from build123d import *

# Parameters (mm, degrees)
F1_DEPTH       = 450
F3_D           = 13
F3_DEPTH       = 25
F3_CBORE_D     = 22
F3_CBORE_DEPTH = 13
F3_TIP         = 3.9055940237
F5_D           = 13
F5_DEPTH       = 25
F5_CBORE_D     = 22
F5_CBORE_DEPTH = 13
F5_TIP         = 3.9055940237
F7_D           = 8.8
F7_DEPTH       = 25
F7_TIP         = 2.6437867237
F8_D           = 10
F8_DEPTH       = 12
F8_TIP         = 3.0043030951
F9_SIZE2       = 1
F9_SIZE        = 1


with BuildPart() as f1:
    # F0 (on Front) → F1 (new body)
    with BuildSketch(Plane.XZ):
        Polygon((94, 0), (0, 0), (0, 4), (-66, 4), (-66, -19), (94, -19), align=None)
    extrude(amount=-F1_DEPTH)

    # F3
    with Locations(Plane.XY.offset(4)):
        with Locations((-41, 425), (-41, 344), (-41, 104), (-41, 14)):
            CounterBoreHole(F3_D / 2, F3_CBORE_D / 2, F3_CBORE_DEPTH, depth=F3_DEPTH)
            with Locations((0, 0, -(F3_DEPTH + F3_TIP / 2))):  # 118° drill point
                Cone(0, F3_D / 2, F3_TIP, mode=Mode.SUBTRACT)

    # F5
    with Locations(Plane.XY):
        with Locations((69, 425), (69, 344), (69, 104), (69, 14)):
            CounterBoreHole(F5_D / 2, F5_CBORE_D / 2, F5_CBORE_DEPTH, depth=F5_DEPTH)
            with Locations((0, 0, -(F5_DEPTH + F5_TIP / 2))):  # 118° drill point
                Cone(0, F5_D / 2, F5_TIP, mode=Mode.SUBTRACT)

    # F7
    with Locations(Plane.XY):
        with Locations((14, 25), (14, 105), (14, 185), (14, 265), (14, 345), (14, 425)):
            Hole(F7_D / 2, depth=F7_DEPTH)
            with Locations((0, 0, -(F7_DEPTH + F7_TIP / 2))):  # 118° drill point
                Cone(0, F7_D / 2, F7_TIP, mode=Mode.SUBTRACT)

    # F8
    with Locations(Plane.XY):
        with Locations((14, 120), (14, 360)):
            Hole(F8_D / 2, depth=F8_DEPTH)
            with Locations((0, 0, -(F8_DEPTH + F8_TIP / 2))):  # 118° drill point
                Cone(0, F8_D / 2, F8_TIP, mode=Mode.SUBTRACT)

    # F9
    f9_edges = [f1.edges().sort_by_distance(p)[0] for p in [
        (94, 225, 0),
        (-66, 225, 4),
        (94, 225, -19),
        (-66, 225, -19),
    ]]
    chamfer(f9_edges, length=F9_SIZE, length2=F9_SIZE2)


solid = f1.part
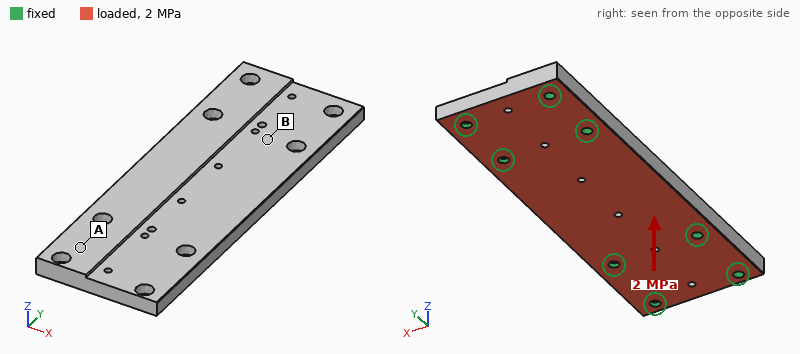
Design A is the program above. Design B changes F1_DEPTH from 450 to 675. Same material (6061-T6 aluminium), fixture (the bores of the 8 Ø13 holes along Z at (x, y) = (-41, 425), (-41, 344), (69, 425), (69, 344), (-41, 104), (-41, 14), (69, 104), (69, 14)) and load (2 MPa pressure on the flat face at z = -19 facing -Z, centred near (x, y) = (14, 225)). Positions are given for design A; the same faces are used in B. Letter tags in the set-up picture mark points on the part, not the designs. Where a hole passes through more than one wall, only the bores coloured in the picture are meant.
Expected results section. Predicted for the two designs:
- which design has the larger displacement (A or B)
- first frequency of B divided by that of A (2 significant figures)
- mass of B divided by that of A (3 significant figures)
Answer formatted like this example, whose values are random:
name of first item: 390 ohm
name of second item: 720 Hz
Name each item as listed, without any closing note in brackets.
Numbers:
which design has the larger displacement: B
first frequency of B divided by that of A: 0.16
mass of B divided by that of A: 1.52
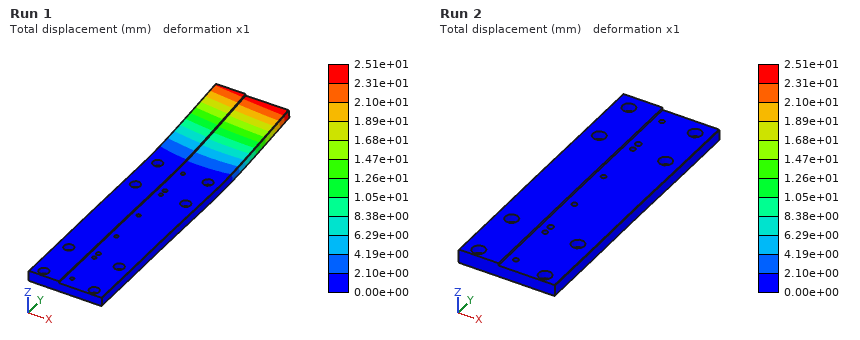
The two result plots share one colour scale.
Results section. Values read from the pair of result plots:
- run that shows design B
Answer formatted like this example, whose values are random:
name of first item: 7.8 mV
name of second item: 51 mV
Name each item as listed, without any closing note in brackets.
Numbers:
run that shows design B: Run 1
